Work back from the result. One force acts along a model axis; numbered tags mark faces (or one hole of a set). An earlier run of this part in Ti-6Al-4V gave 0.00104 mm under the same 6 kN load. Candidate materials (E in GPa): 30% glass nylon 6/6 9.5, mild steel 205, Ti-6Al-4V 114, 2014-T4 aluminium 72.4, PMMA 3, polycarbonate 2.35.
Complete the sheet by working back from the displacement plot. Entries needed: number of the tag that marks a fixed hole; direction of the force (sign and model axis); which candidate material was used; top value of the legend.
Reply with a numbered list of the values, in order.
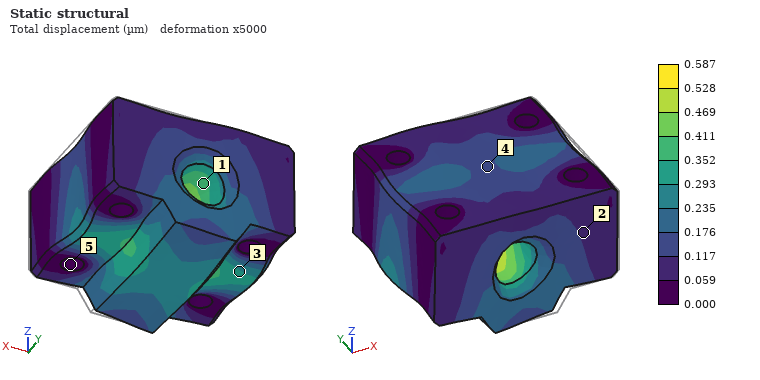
1. 5
2. -X
3. mild steel
4. 0.587 µm
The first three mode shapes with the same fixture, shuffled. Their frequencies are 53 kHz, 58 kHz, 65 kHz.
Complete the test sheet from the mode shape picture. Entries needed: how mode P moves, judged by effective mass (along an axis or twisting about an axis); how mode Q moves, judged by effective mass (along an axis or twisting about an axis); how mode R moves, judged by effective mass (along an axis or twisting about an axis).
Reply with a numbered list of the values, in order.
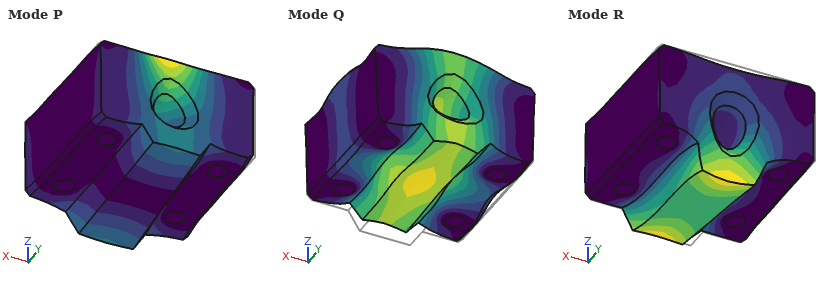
1. along Y
2. along Z
3. along Y
